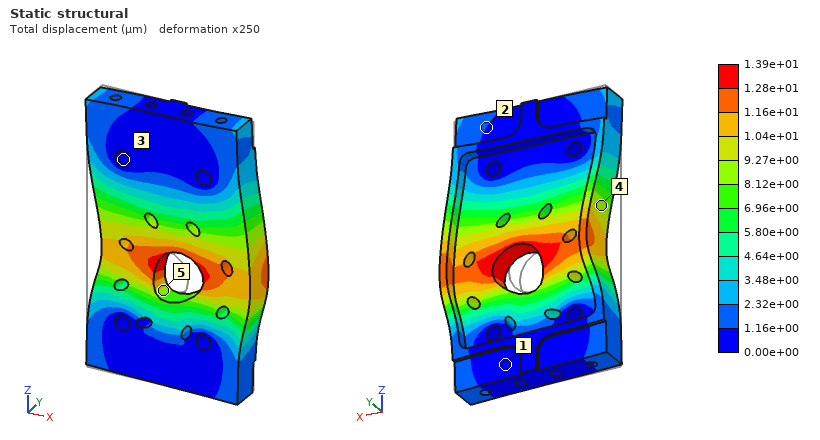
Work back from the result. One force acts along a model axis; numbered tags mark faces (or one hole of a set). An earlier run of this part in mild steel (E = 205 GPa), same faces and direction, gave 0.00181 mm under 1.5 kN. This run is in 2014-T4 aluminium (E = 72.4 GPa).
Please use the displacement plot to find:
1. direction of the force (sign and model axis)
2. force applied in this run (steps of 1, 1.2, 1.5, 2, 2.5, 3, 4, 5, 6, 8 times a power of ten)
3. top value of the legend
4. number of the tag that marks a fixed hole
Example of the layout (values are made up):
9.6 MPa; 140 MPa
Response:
+X; 4 kN; 1.39e+01 µm; 3
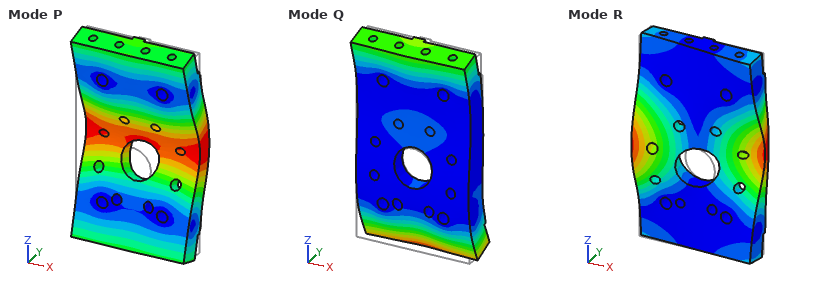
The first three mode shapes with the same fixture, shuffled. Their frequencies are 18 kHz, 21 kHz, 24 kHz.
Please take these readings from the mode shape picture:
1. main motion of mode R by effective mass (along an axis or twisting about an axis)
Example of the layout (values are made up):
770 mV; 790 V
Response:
twisting about Z
